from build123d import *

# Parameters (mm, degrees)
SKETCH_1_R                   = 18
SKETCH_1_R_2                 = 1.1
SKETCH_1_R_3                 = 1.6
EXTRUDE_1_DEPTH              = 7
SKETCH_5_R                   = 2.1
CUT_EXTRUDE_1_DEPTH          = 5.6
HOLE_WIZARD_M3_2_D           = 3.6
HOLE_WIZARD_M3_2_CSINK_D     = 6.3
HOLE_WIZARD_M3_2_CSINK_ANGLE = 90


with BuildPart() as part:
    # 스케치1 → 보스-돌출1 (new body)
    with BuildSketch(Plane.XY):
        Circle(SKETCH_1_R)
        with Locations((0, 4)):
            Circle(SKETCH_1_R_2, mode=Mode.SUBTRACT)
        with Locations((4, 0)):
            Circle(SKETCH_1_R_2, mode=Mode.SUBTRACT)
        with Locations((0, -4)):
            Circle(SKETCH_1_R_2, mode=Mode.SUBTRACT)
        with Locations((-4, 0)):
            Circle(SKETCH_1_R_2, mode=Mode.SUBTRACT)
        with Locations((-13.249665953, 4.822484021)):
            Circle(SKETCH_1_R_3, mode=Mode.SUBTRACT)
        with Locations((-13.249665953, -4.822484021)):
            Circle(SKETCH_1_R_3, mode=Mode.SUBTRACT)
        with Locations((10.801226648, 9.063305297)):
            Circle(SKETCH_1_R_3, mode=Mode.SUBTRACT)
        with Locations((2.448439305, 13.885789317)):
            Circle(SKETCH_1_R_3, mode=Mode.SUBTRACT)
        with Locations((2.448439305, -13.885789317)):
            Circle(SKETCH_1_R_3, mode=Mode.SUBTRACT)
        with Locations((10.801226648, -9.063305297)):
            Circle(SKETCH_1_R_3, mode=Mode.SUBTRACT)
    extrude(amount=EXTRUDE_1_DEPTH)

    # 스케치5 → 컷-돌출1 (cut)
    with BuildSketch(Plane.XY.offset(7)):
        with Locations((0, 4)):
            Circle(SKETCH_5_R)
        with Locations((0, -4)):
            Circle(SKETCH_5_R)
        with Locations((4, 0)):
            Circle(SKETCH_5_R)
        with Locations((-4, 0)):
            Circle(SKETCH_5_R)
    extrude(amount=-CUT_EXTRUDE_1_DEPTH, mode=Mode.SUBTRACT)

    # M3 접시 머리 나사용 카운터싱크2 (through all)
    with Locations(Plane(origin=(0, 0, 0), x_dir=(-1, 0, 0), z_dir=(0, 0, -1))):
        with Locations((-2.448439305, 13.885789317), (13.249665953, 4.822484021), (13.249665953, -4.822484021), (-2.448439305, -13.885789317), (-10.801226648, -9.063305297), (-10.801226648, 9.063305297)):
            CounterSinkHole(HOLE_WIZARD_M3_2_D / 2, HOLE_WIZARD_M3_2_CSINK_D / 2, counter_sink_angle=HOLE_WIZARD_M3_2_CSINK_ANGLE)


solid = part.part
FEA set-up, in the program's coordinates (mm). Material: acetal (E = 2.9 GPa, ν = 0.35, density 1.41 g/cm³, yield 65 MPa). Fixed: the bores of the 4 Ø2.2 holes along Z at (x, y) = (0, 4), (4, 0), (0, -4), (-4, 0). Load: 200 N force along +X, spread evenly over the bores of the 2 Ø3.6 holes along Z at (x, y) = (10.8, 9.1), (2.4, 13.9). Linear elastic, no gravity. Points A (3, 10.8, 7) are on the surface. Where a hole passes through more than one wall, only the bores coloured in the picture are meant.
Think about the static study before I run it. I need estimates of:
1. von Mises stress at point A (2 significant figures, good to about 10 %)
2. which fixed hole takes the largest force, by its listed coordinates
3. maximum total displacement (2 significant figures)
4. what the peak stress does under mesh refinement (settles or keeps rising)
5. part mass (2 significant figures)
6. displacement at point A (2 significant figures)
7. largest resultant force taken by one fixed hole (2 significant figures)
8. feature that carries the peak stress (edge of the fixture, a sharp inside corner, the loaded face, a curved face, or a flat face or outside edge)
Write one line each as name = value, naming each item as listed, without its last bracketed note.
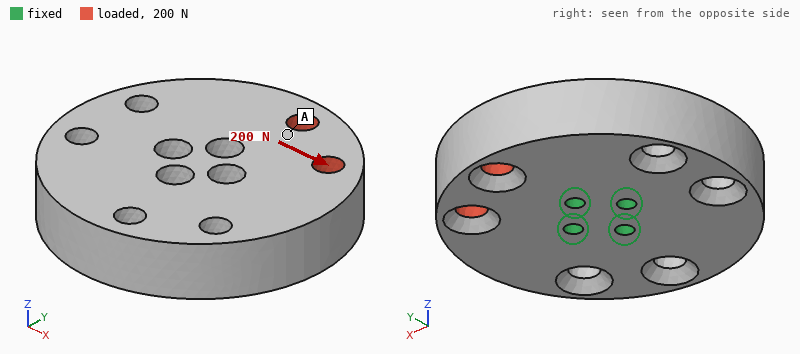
von Mises stress at point A = 3.3 MPa
which fixed hole takes the largest force, by its listed coordinates = (0, 4)
maximum total displacement = 0.12 mm
what the peak stress does under mesh refinement = keeps rising
part mass = 8.9 g
displacement at point A = 0.077 mm
largest resultant force taken by one fixed hole = 190 N
feature that carries the peak stress = edge of the fixture
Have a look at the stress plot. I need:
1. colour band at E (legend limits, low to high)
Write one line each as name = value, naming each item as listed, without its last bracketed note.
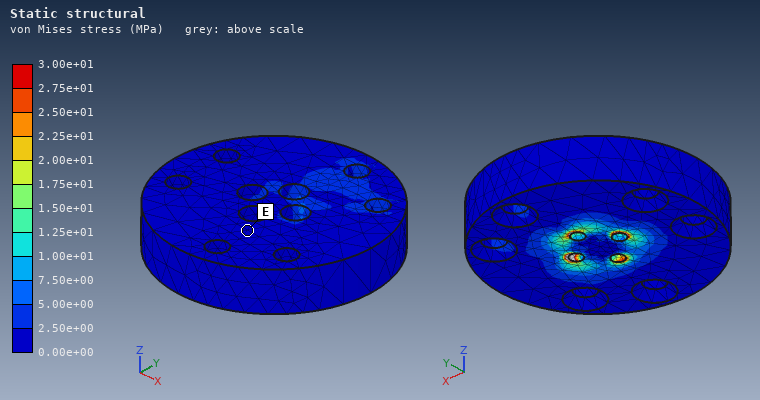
colour band at E = 0.00e+00 to 2.50e+00 MPa
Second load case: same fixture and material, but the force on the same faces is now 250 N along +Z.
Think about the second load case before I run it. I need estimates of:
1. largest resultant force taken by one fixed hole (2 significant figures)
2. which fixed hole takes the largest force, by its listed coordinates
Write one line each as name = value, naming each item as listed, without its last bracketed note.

largest resultant force taken by one fixed hole = 350 N
which fixed hole takes the largest force, by its listed coordinates = (0, 4)
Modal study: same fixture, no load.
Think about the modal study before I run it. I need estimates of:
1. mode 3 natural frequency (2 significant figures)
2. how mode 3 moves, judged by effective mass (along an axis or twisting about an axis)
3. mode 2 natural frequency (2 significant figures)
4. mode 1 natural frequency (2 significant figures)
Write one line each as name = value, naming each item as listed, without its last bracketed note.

mode 3 natural frequency = 3400 Hz
how mode 3 moves, judged by effective mass = twisting about Z
mode 2 natural frequency = 2400 Hz
mode 1 natural frequency = 2400 Hz
